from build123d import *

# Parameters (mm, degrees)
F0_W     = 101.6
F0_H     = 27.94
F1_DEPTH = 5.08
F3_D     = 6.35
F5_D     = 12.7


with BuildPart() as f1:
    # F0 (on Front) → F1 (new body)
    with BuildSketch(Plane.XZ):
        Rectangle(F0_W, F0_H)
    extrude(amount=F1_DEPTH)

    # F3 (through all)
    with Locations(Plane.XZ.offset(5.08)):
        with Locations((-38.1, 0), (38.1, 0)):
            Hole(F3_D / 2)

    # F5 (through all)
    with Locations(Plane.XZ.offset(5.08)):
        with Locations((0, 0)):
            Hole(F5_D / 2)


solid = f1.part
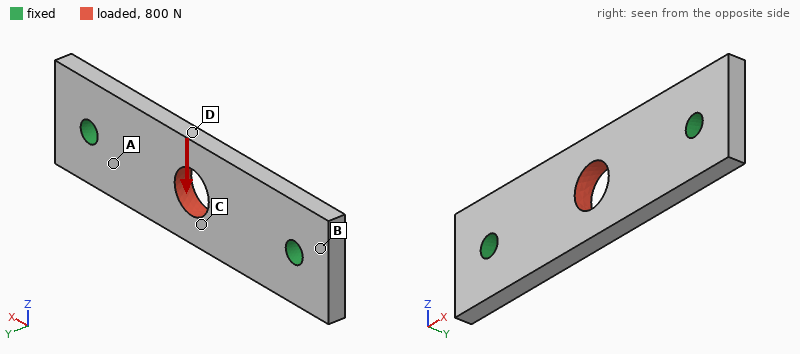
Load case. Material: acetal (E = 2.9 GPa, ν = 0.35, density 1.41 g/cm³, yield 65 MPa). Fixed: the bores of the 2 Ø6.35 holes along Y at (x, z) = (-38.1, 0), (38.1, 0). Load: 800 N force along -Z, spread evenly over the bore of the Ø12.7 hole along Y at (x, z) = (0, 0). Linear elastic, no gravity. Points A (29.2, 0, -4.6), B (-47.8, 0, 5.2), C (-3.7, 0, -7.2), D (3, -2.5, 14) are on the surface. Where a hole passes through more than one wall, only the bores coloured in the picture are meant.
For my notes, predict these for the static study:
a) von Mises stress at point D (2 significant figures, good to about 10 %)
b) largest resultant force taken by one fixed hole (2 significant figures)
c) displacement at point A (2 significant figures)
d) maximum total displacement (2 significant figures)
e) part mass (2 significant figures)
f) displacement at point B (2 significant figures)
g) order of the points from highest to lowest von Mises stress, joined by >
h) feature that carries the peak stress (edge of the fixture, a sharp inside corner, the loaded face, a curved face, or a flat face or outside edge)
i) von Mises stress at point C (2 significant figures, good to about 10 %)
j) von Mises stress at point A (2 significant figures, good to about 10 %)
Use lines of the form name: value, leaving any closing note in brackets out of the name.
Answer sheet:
von Mises stress at point D: 17 MPa
largest resultant force taken by one fixed hole: 400 N
displacement at point A: 0.071 mm
maximum total displacement: 0.27 mm
part mass: 19 g
displacement at point B: 0.048 mm
order of the points from highest to lowest von Mises stress, joined by >: D > C > A > B
feature that carries the peak stress: edge of the fixture
von Mises stress at point C: 8.9 MPa
von Mises stress at point A: 6.6 MPa
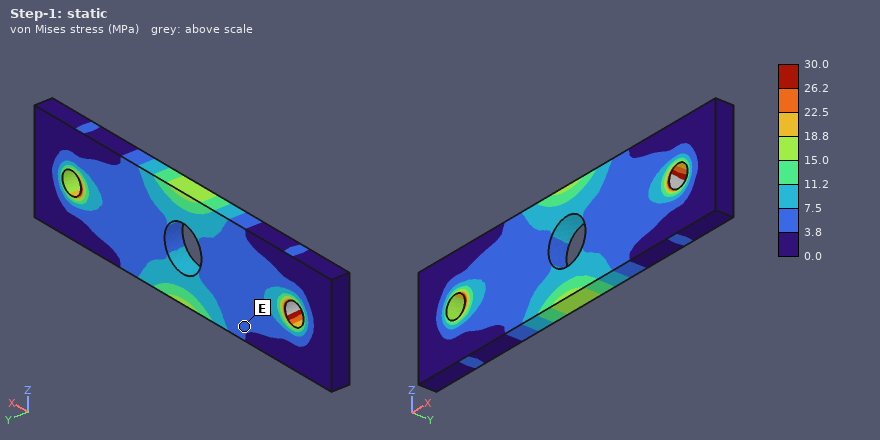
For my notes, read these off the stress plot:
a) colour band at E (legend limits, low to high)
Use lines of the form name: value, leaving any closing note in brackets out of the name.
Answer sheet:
colour band at E: 3.8 to 7.5 MPa
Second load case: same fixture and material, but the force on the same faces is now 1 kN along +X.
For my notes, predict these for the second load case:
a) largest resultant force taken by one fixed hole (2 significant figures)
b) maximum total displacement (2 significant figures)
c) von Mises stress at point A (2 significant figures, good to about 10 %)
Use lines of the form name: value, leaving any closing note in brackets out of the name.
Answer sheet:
largest resultant force taken by one fixed hole: 500 N
maximum total displacement: 56 µm
von Mises stress at point A: 4.6 MPa
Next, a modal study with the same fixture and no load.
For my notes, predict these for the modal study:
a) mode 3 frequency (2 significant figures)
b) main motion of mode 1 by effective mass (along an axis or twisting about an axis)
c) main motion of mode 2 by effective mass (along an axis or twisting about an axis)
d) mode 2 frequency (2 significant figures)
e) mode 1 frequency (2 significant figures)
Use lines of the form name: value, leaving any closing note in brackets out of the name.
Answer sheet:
mode 3 frequency: 3300 Hz
main motion of mode 1 by effective mass: along Y
main motion of mode 2 by effective mass: twisting about X
mode 2 frequency: 2100 Hz
mode 1 frequency: 1300 Hz
